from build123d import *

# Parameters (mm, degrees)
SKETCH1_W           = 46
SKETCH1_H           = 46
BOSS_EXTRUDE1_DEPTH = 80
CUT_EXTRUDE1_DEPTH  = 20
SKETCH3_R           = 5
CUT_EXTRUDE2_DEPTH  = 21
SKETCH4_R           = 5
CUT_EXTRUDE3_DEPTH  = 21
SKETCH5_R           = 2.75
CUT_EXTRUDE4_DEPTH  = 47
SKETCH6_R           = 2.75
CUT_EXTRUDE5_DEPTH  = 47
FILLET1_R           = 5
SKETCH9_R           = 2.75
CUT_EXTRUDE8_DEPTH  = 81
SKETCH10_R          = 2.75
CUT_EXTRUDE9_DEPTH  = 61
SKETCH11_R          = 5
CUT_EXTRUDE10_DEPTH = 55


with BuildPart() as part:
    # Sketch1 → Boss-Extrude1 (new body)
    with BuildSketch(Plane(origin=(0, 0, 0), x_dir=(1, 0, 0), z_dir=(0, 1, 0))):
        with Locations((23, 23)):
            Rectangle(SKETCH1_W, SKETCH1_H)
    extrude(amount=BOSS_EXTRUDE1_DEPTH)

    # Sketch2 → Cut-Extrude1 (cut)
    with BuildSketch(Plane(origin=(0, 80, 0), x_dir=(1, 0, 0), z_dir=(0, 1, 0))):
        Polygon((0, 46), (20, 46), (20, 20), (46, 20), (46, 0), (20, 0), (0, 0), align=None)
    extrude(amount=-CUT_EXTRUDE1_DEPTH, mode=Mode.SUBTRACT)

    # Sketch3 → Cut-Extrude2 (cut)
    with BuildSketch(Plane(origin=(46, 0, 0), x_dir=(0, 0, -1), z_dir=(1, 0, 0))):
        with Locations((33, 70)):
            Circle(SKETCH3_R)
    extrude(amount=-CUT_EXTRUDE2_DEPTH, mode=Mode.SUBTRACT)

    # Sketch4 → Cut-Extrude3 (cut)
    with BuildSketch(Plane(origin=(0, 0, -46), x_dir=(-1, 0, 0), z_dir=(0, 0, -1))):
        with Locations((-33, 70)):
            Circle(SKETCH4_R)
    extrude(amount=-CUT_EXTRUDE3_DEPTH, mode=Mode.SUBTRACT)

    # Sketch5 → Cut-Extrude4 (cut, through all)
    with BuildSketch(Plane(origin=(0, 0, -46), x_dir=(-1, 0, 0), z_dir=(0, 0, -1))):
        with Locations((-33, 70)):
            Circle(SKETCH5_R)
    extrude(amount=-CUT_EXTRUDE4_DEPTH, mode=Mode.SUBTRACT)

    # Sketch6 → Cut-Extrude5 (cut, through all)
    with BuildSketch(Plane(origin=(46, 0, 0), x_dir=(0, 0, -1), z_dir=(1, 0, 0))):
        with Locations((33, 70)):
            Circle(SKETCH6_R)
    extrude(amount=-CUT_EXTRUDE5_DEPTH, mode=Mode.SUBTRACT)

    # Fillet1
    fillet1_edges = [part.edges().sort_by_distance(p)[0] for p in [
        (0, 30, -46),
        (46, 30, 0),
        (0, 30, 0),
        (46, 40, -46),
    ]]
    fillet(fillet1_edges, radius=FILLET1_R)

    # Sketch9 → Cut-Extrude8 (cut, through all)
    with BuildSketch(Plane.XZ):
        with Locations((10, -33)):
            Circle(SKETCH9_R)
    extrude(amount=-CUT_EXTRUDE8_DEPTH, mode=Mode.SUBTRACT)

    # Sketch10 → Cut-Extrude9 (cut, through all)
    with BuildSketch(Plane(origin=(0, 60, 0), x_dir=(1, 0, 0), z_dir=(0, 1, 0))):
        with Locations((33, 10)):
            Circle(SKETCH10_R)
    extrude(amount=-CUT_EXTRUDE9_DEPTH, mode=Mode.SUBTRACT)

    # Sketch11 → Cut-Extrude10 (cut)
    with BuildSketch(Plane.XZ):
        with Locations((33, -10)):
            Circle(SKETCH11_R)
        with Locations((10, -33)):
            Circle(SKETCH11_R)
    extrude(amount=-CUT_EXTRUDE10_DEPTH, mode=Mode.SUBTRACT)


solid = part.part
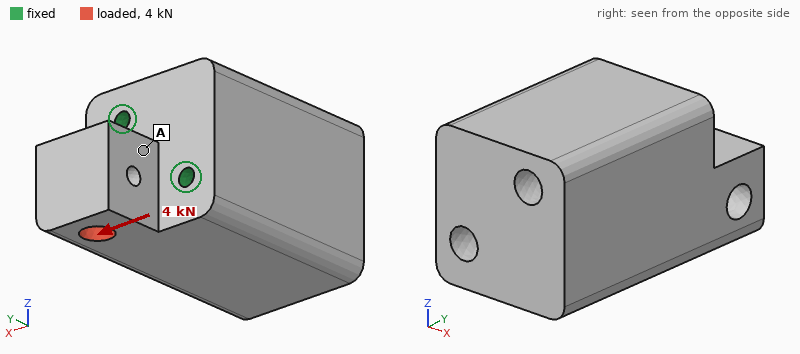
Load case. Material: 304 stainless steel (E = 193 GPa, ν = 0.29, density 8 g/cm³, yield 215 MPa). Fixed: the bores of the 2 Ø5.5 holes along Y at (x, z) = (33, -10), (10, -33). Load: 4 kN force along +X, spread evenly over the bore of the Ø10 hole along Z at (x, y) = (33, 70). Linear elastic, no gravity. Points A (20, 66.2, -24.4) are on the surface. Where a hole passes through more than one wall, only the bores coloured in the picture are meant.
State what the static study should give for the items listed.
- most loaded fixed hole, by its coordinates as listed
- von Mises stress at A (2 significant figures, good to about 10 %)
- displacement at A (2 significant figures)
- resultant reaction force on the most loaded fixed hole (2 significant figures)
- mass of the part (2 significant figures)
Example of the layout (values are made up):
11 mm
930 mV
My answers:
(10, -33)
20 MPa
8.6 µm
4.1 kN
1.0 kg
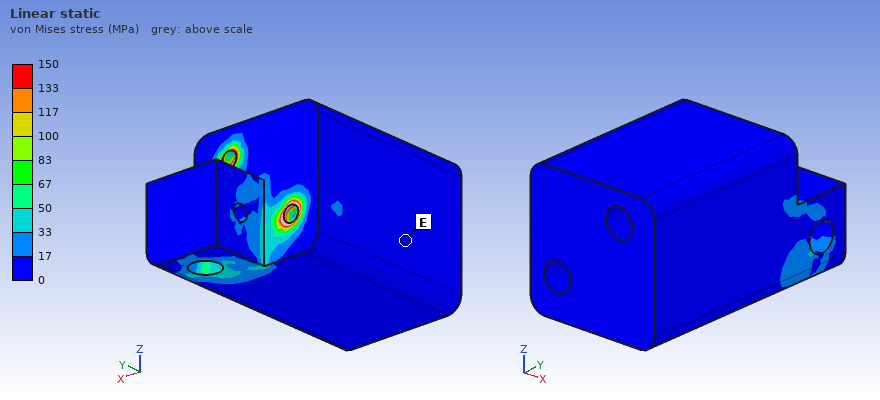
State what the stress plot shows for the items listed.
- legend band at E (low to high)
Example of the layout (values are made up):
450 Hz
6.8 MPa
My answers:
0 to 17 MPa
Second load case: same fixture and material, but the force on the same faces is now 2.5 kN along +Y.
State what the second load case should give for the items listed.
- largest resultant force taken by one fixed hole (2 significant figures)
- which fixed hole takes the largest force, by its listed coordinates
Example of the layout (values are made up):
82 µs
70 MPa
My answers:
1.7 kN
(10, -33)
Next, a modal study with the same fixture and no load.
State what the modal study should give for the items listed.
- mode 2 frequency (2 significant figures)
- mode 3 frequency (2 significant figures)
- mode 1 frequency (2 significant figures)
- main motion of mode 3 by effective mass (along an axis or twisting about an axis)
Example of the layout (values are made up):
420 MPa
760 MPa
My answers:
3800 Hz
7700 Hz
1000 Hz
twisting about Y
